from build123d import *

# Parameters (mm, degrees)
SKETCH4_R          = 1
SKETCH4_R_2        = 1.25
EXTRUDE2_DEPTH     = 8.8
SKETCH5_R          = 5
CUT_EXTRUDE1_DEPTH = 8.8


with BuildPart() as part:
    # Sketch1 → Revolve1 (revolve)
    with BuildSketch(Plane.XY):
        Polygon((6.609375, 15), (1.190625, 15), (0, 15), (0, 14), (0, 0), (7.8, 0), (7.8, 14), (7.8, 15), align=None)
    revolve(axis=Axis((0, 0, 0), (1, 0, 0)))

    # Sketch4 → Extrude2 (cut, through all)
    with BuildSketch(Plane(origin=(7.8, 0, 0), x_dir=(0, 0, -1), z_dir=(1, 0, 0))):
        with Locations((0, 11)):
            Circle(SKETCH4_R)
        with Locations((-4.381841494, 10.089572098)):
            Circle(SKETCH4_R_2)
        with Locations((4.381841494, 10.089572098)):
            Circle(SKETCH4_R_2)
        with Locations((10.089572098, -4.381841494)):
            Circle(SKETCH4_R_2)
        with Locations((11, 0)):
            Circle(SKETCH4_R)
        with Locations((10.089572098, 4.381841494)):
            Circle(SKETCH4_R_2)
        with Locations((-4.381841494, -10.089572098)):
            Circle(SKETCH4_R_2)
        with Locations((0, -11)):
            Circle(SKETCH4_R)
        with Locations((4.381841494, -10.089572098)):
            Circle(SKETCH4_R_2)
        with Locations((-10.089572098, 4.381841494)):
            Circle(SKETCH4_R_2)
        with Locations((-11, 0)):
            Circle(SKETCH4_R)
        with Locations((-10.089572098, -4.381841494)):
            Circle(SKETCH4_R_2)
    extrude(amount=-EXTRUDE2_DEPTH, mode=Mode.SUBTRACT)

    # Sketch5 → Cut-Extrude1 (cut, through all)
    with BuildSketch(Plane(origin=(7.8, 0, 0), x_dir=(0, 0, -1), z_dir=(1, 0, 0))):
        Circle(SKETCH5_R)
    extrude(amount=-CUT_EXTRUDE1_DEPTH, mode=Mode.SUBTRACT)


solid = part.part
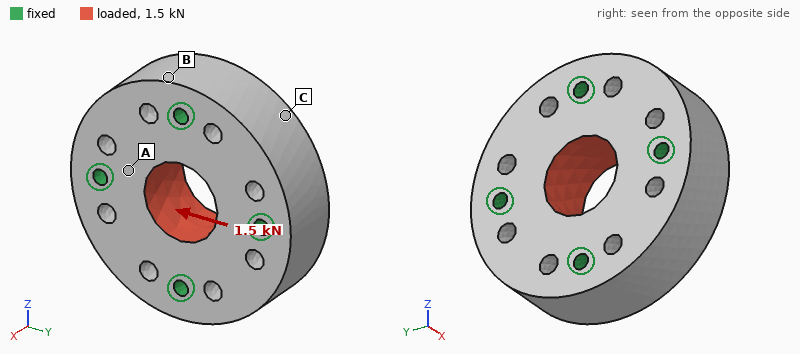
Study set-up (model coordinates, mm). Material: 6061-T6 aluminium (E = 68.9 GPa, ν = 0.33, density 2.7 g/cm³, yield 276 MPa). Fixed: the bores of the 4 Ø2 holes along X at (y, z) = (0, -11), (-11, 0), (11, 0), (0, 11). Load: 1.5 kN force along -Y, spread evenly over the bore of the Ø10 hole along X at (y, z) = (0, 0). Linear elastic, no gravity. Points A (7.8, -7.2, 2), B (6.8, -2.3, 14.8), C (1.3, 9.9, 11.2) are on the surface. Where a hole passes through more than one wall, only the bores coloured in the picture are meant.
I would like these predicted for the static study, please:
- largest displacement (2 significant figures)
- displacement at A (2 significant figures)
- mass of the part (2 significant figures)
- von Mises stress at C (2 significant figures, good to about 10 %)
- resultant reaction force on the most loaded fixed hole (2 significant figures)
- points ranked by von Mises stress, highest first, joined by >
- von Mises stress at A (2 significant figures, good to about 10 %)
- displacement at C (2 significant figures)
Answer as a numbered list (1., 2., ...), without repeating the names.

1. 1.2 µm
2. 0.59 µm
3. 12 g
4. 3.6 MPa
5. 460 N
6. A > C > B
7. 9.4 MPa
8. 0.57 µm
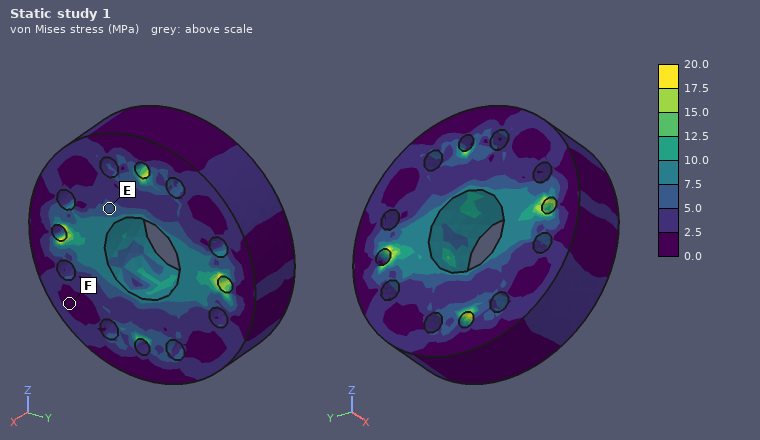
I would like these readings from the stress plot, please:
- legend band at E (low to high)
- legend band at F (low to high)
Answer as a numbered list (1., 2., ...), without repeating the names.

1. 5.0 to 7.5 MPa
2. 0.0 to 2.5 MPa
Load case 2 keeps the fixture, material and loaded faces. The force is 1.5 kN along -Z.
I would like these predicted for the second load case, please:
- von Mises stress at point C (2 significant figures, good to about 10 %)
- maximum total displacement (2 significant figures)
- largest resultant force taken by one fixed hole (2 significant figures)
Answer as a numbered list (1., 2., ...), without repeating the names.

1. 3.7 MPa
2. 1.2 µm
3. 460 N
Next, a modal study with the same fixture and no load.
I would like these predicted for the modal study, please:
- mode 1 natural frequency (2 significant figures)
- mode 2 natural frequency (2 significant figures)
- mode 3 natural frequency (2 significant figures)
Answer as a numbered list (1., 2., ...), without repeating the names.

1. 54 kHz
2. 58 kHz
3. 58 kHz
